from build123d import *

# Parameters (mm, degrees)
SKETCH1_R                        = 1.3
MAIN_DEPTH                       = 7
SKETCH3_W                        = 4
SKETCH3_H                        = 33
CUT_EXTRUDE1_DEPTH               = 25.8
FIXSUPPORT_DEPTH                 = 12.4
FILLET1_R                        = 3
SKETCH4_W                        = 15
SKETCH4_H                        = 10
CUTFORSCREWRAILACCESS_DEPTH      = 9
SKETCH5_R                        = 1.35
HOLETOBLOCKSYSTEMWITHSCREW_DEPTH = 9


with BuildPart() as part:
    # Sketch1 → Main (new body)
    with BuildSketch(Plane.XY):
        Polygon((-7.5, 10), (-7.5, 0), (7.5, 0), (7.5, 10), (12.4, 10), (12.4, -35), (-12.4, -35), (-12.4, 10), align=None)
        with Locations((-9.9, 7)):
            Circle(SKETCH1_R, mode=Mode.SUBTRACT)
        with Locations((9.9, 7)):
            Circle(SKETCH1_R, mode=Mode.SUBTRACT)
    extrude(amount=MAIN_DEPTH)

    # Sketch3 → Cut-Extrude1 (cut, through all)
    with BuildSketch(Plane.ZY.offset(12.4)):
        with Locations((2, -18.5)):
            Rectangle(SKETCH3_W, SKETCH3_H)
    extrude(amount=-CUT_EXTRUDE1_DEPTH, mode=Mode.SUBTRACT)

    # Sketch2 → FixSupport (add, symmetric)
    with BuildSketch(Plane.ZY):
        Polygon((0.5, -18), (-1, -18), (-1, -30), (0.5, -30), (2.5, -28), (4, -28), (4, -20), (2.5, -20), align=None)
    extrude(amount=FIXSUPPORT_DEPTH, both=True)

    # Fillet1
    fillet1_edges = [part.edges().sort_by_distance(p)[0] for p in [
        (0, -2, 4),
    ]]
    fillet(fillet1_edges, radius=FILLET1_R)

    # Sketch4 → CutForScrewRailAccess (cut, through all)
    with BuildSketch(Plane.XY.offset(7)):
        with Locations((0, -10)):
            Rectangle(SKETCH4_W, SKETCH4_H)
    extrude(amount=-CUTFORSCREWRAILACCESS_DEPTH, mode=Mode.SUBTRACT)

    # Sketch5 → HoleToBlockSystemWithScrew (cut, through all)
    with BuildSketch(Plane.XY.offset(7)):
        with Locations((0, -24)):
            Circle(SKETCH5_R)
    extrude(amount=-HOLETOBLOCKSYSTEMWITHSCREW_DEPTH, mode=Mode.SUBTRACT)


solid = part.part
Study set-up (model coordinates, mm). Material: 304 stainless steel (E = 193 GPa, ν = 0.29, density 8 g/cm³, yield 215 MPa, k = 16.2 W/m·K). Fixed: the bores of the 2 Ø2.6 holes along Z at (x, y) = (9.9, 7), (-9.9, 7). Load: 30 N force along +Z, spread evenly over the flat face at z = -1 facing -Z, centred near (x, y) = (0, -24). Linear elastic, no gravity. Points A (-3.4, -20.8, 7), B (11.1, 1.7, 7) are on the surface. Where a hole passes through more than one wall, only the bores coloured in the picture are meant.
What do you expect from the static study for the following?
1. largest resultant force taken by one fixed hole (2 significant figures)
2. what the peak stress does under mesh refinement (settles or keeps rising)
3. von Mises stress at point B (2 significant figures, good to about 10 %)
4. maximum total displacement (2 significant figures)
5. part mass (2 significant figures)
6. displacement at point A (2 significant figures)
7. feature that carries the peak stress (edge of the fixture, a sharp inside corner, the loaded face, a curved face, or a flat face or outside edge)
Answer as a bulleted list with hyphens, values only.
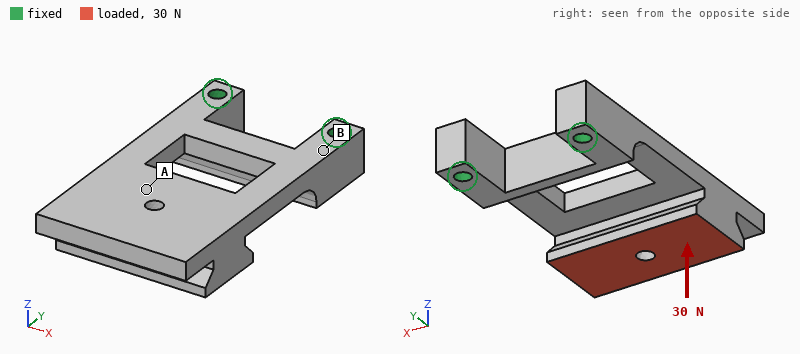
- 15 N
- keeps rising
- 11 MPa
- 43 µm
- 34 g
- 21 µm
- a sharp inside corner
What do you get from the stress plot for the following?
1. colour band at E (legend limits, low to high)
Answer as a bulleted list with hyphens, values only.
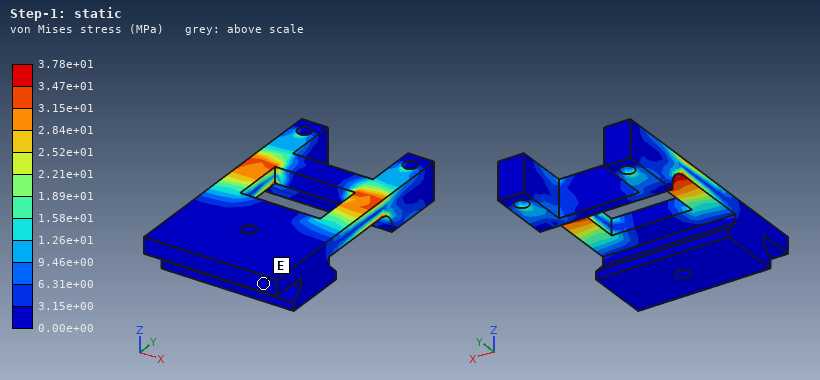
- 0.00e+00 to 3.15e+00 MPa
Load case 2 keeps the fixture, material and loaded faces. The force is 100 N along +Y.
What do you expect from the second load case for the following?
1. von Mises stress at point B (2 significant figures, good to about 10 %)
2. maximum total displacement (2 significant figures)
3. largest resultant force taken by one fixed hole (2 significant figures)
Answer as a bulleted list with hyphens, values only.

- 5.1 MPa
- 62 µm
- 50 N
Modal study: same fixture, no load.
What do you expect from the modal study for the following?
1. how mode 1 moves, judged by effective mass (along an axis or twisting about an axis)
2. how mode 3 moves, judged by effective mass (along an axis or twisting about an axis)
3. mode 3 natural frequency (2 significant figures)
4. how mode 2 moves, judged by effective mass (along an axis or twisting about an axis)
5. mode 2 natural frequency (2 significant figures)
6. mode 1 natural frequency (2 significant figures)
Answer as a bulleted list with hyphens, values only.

- along Z
- along X
- 5000 Hz
- along X
- 3700 Hz
- 1100 Hz
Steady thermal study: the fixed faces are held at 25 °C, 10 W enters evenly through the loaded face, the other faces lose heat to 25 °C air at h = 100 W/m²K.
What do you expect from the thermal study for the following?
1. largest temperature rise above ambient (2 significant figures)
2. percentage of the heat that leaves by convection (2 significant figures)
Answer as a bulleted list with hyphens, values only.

- 72 K
- 93 %
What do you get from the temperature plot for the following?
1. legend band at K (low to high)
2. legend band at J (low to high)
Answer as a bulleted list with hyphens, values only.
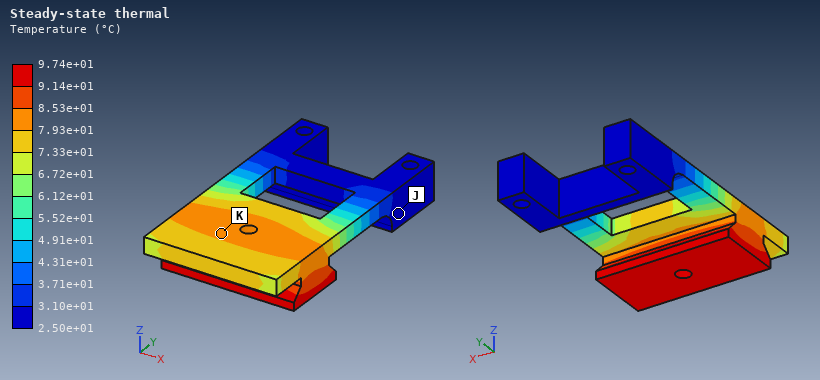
- 7.93e+01 to 8.53e+01 °C
- 2.50e+01 to 3.10e+01 °C
